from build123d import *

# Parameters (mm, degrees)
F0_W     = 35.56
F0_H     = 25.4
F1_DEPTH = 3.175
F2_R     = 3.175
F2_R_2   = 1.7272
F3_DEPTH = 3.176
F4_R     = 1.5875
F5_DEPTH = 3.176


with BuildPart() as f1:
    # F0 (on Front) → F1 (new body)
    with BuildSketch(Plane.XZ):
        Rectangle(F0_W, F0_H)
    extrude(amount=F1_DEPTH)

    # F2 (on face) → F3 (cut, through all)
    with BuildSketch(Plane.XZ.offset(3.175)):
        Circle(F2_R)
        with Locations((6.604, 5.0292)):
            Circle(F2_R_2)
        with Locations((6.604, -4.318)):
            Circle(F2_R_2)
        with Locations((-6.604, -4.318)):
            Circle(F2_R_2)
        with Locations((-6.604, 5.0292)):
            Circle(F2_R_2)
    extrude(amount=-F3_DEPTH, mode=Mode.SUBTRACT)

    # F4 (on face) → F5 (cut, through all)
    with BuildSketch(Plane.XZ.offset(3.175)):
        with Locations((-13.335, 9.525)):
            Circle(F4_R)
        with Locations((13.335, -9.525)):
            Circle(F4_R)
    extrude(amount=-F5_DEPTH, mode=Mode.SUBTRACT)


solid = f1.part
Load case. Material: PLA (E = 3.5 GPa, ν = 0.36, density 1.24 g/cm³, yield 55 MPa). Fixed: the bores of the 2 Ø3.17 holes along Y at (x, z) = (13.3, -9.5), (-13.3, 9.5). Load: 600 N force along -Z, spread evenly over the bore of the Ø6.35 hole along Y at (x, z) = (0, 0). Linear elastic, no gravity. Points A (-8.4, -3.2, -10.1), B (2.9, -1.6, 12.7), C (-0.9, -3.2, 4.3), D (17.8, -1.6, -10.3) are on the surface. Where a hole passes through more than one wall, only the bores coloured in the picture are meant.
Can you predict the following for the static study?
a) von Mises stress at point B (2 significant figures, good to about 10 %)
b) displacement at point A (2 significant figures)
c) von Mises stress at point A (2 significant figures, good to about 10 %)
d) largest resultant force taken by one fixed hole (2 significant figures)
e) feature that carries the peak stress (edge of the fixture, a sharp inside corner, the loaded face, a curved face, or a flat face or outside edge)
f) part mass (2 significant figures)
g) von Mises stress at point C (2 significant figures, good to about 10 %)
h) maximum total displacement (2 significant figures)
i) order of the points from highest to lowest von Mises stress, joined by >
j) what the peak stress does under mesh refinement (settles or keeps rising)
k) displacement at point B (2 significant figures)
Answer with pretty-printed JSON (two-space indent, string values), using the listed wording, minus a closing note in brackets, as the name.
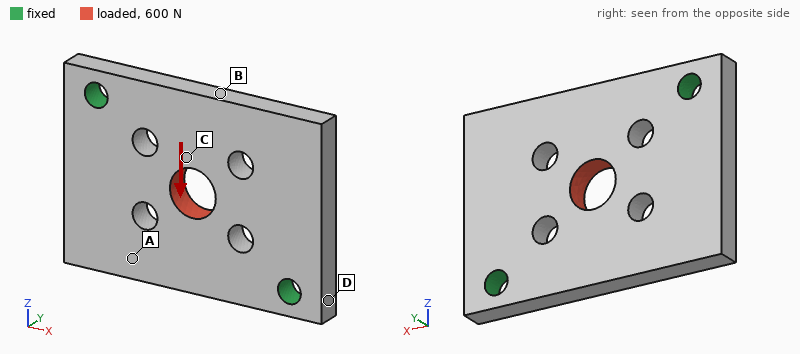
{
  "von Mises stress at point B": "14 MPa",
  "displacement at point A": "57 µm",
  "von Mises stress at point A": "6.0 MPa",
  "largest resultant force taken by one fixed hole": "300 N",
  "feature that carries the peak stress": "edge of the fixture",
  "part mass": "3.2 g",
  "von Mises stress at point C": "9.3 MPa",
  "maximum total displacement": "86 µm",
  "order of the points from highest to lowest von Mises stress, joined by >": "B > C > A > D",
  "what the peak stress does under mesh refinement": "keeps rising",
  "displacement at point B": "72 µm"
}
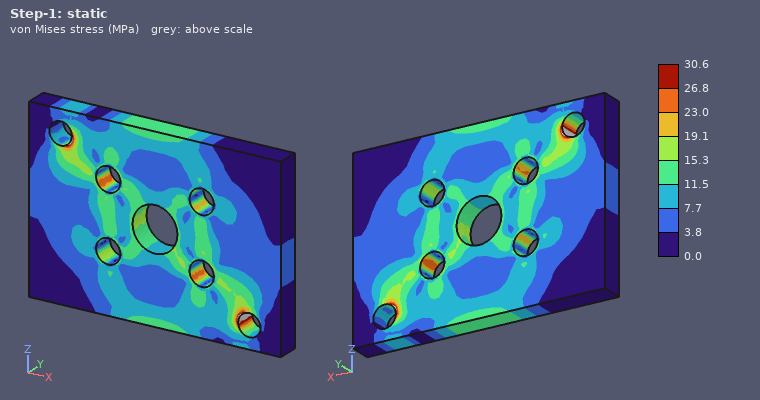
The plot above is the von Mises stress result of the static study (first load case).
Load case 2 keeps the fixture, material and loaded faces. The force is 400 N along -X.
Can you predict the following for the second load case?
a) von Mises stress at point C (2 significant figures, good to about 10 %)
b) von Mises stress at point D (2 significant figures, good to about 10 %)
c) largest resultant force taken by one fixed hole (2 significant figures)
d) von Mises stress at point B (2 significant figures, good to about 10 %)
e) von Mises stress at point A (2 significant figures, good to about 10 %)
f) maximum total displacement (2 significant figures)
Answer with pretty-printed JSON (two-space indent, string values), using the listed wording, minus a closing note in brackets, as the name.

{
  "von Mises stress at point C": "5.9 MPa",
  "von Mises stress at point D": "2.3 MPa",
  "largest resultant force taken by one fixed hole": "200 N",
  "von Mises stress at point B": "5.9 MPa",
  "von Mises stress at point A": "2.9 MPa",
  "maximum total displacement": "44 µm"
}
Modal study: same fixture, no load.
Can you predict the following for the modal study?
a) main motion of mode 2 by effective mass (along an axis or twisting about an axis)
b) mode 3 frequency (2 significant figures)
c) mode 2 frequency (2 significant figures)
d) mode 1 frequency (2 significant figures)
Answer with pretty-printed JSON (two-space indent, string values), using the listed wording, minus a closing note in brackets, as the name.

{
  "main motion of mode 2 by effective mass": "along Y",
  "mode 3 frequency": "5700 Hz",
  "mode 2 frequency": "2700 Hz",
  "mode 1 frequency": "2100 Hz"
}
